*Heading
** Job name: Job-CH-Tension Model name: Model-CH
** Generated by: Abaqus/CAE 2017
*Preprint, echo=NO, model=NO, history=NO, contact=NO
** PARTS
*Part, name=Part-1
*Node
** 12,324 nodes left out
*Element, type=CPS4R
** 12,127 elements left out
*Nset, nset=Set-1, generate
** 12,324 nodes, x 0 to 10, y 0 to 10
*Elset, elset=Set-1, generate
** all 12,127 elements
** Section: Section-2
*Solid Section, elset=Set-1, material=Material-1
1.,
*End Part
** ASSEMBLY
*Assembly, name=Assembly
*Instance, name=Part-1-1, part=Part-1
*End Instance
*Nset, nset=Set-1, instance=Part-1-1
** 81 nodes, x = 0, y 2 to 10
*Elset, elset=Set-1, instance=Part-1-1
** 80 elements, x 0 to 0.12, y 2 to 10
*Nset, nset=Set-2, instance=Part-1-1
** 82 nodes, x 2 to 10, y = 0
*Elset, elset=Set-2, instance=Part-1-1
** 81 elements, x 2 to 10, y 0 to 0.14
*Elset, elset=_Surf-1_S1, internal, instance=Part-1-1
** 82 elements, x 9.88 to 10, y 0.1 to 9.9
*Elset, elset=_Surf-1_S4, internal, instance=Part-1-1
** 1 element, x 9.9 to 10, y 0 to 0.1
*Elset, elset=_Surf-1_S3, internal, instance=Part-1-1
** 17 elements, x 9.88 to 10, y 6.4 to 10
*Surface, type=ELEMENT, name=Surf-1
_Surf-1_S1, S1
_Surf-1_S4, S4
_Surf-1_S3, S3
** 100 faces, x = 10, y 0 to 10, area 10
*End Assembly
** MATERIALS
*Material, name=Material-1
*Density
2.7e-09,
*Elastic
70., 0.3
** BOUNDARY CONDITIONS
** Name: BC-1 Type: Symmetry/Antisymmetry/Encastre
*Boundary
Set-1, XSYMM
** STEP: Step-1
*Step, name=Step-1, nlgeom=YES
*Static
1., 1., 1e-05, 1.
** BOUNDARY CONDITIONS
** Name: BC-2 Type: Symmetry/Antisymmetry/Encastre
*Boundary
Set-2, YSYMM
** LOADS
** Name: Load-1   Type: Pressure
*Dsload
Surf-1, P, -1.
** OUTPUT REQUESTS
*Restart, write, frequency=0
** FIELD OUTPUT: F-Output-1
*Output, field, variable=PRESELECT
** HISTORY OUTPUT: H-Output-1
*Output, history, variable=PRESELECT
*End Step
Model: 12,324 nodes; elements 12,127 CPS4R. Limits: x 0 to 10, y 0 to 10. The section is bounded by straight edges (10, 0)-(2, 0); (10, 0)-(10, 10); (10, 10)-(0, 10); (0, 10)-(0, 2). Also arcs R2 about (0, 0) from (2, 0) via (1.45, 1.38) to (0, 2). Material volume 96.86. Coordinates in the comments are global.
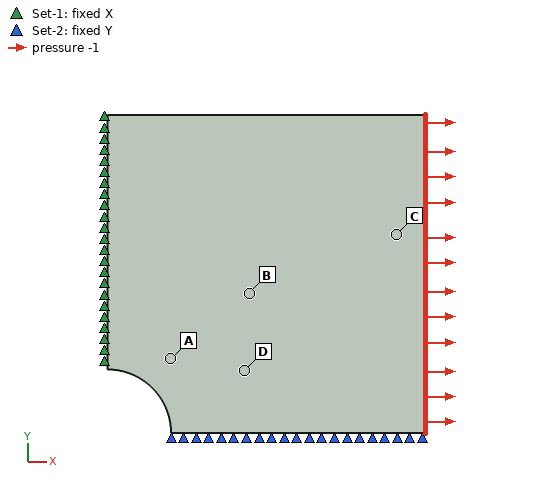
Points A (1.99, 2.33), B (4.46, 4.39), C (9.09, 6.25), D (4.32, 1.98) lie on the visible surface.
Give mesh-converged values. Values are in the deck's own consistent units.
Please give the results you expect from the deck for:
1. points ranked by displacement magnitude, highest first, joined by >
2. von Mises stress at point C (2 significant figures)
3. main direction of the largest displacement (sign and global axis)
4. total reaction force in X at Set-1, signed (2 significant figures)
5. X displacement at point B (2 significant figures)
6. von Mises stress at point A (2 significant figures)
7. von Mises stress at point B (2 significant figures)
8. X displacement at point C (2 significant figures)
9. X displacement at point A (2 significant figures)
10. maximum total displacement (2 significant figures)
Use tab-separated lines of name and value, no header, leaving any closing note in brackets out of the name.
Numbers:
points ranked by displacement magnitude, highest first, joined by >	C > D > B > A
von Mises stress at point C	1.0
main direction of the largest displacement	+X
total reaction force in X at Set-1, signed	-9.9
X displacement at point B	0.076
von Mises stress at point A	1.5
von Mises stress at point B	1.2
X displacement at point C	0.14
X displacement at point A	0.049
maximum total displacement	0.17
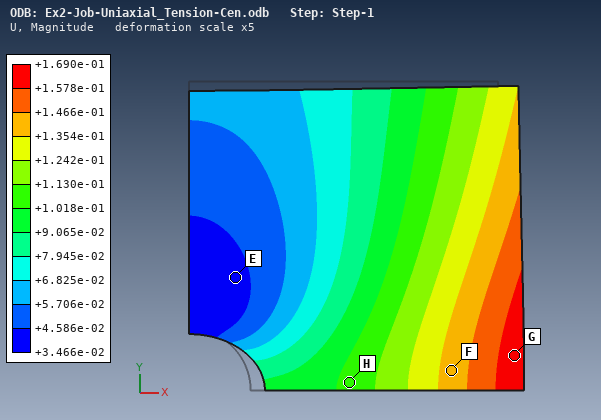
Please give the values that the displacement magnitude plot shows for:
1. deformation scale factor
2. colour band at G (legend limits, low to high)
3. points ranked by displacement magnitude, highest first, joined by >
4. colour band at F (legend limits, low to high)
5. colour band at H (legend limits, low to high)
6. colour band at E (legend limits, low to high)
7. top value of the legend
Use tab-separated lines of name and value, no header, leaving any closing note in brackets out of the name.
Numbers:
deformation scale factor	5
colour band at G	+1.578e-01 to +1.690e-01
points ranked by displacement magnitude, highest first, joined by >	G > F > H > E
colour band at F	+1.354e-01 to +1.466e-01
colour band at H	+1.018e-01 to +1.130e-01
colour band at E	+3.466e-02 to +4.586e-02
top value of the legend	+1.690e-01
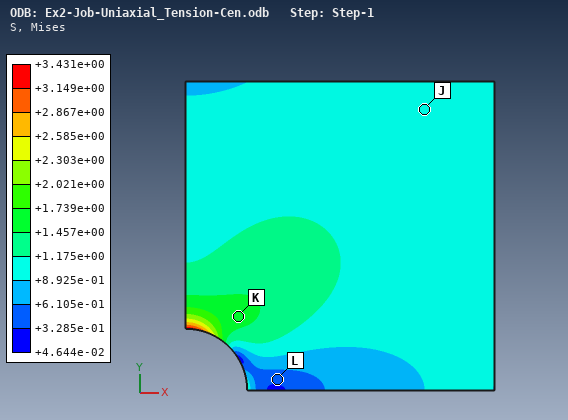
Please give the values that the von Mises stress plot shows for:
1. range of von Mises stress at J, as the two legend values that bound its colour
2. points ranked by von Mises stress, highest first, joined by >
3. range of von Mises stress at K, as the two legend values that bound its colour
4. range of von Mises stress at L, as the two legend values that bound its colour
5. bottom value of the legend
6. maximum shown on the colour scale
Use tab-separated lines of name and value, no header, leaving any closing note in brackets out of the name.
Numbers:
range of von Mises stress at J, as the two legend values that bound its colour	+8.925e-01 to +1.175e+00
points ranked by von Mises stress, highest first, joined by >	K > J > L
range of von Mises stress at K, as the two legend values that bound its colour	+1.457e+00 to +1.739e+00
range of von Mises stress at L, as the two legend values that bound its colour	+3.285e-01 to +6.105e-01
bottom value of the legend	+4.644e-02
maximum shown on the colour scale	+3.431e+00
